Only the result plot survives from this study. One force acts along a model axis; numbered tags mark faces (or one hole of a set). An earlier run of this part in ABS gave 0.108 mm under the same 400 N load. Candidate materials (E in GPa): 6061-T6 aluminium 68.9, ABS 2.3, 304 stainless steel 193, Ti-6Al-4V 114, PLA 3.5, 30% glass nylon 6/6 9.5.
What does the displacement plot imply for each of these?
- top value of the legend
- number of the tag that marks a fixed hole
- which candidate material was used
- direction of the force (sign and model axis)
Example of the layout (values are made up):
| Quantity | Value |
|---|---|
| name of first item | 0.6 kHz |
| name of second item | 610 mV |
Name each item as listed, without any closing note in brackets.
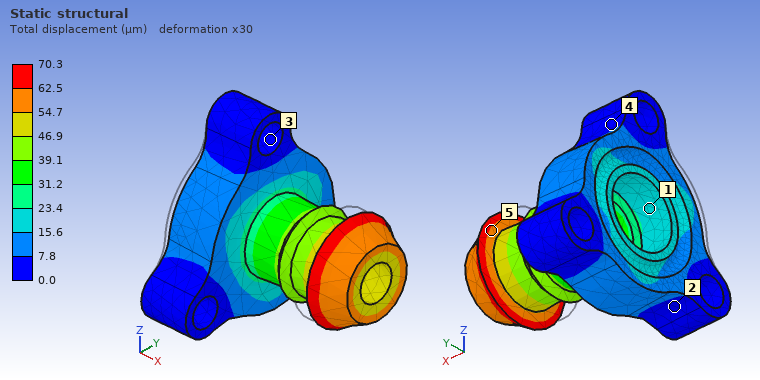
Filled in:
| Quantity | Value |
|---|---|
| top value of the legend | 70.3 µm |
| number of the tag that marks a fixed hole | 3 |
| which candidate material was used | PLA |
| direction of the force | +X |
